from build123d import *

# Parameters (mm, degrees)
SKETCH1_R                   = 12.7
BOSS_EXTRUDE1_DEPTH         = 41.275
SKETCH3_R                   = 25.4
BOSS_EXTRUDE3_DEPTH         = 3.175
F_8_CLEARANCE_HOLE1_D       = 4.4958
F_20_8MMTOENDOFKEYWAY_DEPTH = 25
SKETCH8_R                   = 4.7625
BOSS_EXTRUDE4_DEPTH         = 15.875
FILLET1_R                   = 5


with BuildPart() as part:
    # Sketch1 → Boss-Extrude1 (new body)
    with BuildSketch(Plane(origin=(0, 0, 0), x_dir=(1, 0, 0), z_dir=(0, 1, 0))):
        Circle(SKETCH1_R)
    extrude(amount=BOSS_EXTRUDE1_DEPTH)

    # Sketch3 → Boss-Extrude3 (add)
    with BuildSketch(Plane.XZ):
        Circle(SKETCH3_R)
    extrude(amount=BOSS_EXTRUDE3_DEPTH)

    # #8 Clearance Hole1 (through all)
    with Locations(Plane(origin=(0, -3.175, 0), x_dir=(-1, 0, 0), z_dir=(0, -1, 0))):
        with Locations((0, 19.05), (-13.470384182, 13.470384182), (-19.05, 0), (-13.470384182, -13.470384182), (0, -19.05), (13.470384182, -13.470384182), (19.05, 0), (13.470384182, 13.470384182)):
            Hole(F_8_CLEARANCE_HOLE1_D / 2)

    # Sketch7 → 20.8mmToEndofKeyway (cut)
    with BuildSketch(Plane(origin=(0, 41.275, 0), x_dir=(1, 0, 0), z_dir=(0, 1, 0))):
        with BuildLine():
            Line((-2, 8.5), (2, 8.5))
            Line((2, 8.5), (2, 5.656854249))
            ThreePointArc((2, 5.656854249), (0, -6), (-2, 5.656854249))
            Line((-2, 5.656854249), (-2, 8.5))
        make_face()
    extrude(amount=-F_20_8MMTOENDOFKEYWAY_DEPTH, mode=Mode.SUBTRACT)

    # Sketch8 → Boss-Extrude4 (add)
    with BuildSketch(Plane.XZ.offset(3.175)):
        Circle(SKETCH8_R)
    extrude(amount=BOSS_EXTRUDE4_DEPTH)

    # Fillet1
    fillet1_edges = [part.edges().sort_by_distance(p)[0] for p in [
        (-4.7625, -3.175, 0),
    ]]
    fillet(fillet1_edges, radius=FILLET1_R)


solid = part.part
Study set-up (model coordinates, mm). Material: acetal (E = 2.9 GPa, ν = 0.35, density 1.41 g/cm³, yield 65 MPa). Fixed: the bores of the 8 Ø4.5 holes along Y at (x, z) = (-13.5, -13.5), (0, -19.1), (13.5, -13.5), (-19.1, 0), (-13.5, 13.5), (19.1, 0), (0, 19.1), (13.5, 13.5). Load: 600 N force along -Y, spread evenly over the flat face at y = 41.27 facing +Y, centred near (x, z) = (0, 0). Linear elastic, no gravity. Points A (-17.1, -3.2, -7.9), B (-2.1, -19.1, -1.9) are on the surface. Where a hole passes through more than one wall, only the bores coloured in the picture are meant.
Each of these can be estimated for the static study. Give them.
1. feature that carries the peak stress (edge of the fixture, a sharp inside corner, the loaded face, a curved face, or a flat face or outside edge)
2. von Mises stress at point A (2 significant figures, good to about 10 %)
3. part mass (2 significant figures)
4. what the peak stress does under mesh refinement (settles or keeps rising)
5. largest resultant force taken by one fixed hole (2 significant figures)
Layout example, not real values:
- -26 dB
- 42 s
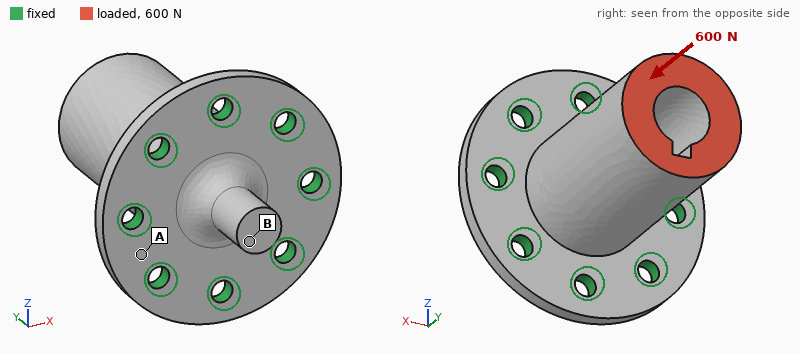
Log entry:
- edge of the fixture
- 2.8 MPa
- 36 g
- keeps rising
- 84 N
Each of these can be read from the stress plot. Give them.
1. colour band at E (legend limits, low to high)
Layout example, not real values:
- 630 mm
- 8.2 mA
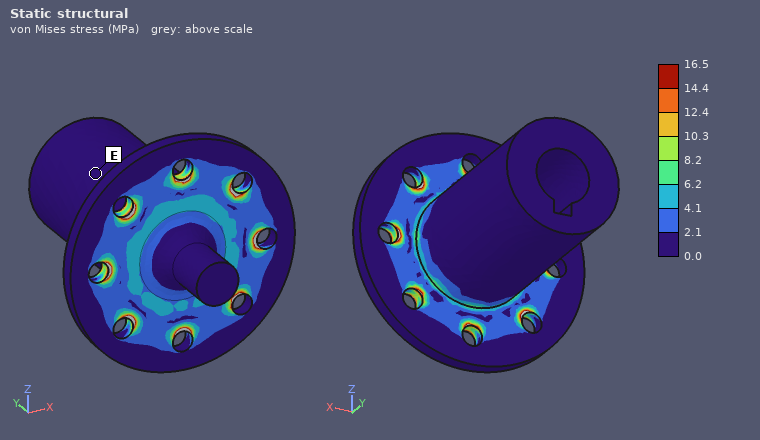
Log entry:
- 0.0 to 2.1 MPa
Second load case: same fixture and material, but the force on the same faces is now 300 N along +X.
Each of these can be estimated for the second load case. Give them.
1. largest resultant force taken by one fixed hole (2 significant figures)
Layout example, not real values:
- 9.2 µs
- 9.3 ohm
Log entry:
- 220 N
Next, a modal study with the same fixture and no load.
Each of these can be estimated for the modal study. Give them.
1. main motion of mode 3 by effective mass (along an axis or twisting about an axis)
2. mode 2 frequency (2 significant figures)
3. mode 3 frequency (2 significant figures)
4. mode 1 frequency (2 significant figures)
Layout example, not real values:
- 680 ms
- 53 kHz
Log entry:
- along Y
- 1500 Hz
- 3500 Hz
- 1500 Hz
